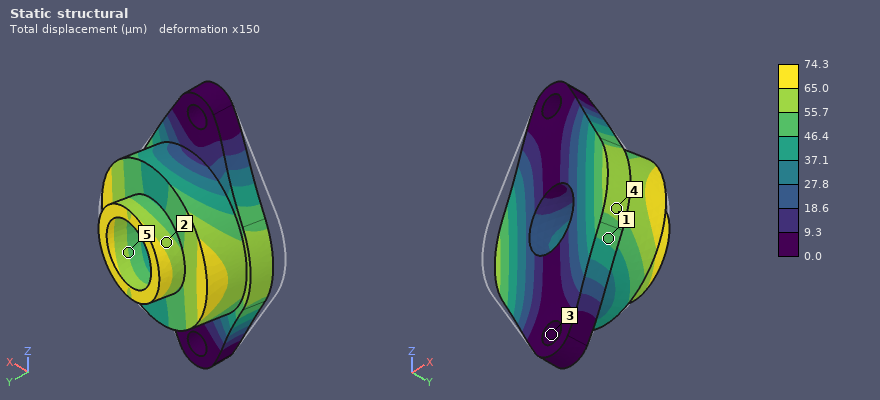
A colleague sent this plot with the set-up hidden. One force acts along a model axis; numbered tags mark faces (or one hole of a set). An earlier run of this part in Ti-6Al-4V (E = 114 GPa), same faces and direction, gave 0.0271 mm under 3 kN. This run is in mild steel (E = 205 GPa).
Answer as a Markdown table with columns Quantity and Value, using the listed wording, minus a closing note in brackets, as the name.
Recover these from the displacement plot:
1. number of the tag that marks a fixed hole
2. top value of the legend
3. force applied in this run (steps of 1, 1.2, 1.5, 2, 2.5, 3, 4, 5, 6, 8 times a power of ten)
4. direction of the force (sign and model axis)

| Quantity | Value |
|---|---|
| number of the tag that marks a fixed hole | 3 |
| top value of the legend | 74.3 µm |
| force applied in this run | 15 kN |
| direction of the force | +X |
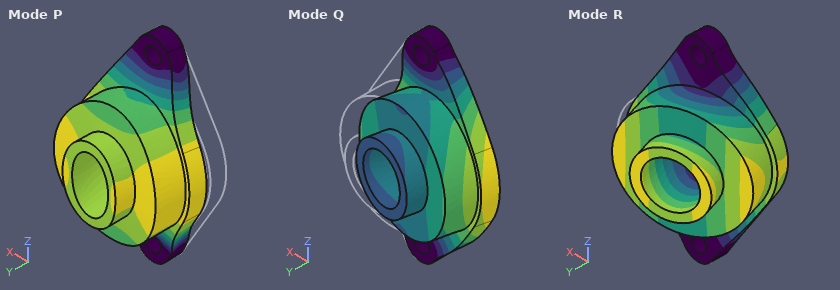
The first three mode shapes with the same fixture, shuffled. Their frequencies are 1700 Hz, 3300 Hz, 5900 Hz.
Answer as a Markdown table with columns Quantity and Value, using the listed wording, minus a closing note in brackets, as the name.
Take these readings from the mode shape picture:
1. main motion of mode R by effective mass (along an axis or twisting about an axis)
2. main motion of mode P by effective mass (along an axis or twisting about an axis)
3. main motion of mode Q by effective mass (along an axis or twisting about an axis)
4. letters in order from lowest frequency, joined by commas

| Quantity | Value |
|---|---|
| main motion of mode R by effective mass | along X |
| main motion of mode P by effective mass | along Y |
| main motion of mode Q by effective mass | along X |
| letters in order from lowest frequency, joined by commas | R, P, Q |
